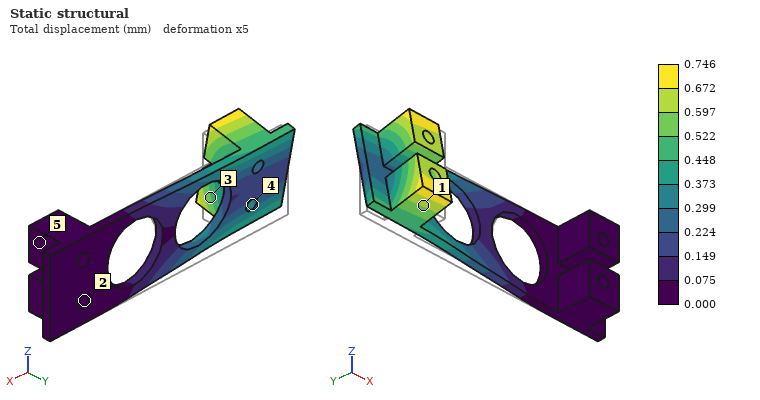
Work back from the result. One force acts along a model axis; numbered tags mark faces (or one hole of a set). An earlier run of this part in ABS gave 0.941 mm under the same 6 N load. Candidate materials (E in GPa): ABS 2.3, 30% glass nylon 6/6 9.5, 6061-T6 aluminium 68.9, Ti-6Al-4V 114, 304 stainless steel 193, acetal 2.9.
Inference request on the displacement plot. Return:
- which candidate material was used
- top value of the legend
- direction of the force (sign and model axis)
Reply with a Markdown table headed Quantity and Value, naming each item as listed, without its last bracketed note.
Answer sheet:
| Quantity | Value |
|---|---|
| which candidate material was used | acetal |
| top value of the legend | 0.746 mm |
| direction of the force | +Z |
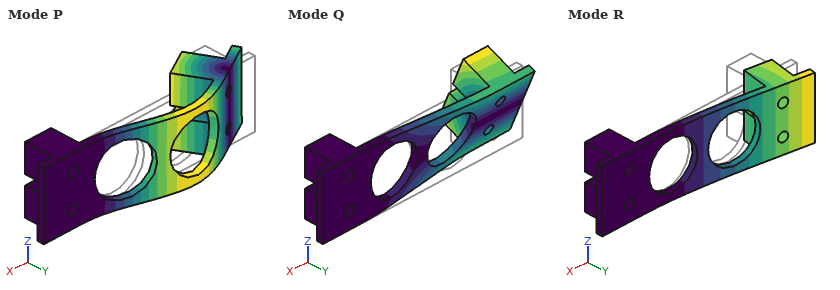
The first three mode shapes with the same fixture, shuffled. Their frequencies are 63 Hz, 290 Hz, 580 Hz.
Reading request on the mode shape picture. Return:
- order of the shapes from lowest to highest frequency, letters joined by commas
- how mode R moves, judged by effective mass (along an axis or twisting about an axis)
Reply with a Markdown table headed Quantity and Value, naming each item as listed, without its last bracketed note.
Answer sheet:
| Quantity | Value |
|---|---|
| order of the shapes from lowest to highest frequency, letters joined by commas | R, Q, P |
| how mode R moves, judged by effective mass | along Y |
